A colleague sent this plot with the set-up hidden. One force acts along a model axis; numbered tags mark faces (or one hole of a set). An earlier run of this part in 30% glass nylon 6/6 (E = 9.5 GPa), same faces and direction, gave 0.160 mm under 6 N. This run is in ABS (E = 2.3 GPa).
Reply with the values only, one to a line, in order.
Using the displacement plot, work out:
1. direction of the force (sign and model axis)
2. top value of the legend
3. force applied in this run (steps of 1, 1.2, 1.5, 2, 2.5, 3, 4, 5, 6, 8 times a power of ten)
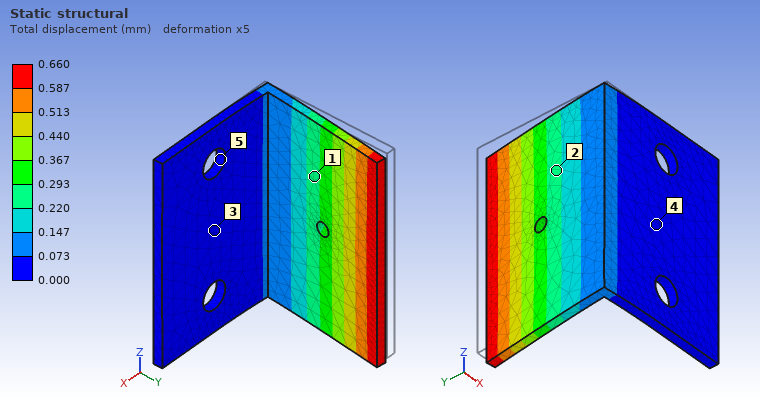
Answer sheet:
+X
0.660 mm
6 N
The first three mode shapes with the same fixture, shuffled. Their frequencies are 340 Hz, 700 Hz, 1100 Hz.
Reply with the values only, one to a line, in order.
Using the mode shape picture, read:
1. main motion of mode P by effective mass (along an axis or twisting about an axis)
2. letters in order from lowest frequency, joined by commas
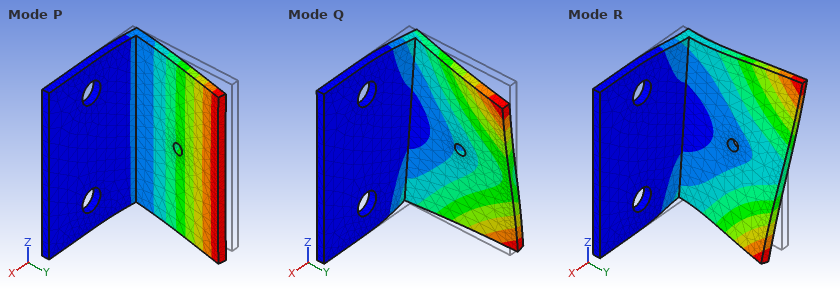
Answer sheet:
along X
P, Q, R
